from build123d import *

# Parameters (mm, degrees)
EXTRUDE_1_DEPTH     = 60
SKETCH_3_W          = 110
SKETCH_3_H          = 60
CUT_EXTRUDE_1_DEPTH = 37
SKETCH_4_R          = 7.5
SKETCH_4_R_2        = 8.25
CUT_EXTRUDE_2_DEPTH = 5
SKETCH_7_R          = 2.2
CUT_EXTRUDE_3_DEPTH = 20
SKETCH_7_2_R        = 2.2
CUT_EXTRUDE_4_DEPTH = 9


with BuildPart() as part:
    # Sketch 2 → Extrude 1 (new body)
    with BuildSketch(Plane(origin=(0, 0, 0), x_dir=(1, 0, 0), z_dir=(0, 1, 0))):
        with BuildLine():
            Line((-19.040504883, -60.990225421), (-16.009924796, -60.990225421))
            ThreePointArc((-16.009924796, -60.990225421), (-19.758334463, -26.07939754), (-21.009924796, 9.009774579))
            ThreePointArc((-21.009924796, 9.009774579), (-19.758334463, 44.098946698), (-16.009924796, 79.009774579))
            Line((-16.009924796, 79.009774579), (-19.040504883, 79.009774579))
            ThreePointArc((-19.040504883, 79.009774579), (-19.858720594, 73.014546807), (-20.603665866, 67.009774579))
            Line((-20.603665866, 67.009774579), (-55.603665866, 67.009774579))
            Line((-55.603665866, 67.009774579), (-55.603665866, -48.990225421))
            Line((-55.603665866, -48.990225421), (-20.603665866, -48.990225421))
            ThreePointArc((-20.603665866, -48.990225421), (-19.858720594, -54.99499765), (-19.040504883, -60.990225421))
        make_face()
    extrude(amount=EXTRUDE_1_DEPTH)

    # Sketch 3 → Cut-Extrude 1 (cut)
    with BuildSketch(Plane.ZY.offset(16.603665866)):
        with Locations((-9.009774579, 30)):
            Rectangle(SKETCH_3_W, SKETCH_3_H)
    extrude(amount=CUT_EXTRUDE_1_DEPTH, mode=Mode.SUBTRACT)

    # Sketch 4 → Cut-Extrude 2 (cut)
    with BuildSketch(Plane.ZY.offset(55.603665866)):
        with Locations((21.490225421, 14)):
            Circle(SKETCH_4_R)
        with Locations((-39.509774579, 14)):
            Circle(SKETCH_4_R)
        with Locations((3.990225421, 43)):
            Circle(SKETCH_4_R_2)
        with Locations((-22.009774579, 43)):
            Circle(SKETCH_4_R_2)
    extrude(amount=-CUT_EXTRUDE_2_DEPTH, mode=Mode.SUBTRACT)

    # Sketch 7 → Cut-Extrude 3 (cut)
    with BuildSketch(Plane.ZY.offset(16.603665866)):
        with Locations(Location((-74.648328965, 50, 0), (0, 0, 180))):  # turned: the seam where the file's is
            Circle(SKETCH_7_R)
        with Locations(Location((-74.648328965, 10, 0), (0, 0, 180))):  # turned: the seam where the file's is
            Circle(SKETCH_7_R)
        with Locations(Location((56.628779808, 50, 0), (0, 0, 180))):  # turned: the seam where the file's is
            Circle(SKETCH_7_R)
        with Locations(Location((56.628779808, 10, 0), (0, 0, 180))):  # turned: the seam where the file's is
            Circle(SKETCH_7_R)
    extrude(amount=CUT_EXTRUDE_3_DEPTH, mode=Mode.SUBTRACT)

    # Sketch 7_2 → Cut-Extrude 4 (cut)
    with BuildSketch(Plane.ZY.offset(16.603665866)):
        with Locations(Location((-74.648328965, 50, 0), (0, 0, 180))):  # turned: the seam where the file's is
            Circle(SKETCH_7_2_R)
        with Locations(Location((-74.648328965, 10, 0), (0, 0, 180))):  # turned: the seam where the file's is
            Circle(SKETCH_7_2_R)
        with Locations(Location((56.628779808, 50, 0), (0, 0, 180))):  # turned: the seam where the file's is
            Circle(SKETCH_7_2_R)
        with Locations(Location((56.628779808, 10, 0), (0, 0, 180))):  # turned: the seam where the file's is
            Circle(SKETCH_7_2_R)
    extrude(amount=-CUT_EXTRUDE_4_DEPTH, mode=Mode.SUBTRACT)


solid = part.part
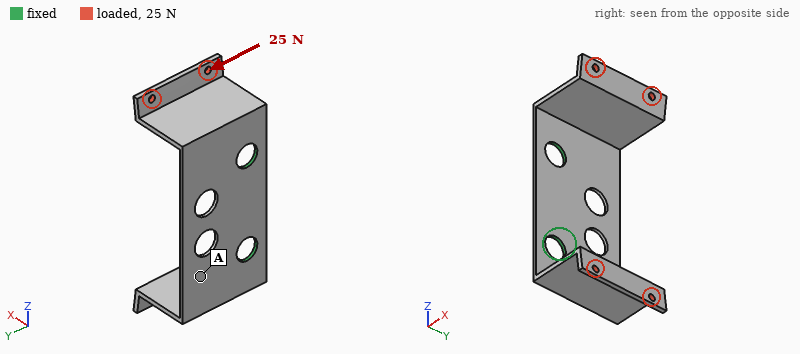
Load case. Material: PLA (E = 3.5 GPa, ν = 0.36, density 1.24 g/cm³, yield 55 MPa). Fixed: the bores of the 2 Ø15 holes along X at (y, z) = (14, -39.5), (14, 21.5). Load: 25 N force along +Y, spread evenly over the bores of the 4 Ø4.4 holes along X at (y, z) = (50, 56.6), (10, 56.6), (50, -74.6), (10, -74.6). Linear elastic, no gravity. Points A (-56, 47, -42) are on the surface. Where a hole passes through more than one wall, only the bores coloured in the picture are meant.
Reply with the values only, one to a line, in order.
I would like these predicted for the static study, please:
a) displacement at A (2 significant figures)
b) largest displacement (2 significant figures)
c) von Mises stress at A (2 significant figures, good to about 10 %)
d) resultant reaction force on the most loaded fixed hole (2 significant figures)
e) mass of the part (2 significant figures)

0.51 mm
1.8 mm
1.7 MPa
15 N
36 g
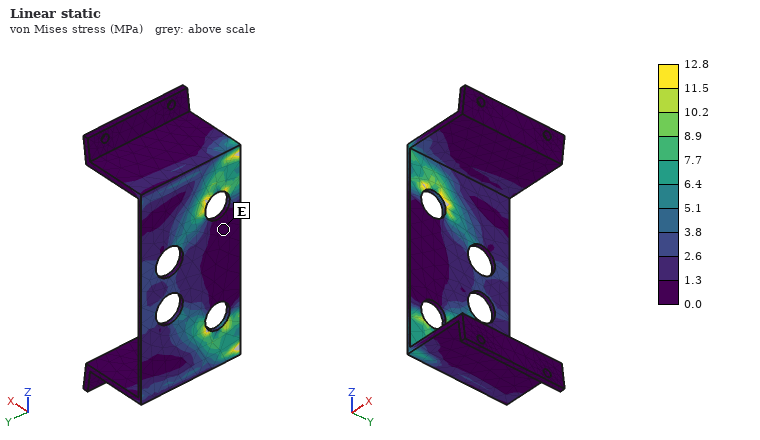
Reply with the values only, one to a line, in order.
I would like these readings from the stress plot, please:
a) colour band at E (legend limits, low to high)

0.0 to 1.3 MPa
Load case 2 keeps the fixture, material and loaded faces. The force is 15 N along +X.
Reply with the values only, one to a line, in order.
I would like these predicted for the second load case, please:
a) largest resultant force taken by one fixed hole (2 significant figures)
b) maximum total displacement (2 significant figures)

7.6 N
1.6 mm
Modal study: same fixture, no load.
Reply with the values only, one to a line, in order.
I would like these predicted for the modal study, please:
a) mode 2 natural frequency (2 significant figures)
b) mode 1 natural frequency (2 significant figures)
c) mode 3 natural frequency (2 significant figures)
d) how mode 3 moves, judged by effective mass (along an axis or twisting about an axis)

120 Hz
120 Hz
190 Hz
along Y
